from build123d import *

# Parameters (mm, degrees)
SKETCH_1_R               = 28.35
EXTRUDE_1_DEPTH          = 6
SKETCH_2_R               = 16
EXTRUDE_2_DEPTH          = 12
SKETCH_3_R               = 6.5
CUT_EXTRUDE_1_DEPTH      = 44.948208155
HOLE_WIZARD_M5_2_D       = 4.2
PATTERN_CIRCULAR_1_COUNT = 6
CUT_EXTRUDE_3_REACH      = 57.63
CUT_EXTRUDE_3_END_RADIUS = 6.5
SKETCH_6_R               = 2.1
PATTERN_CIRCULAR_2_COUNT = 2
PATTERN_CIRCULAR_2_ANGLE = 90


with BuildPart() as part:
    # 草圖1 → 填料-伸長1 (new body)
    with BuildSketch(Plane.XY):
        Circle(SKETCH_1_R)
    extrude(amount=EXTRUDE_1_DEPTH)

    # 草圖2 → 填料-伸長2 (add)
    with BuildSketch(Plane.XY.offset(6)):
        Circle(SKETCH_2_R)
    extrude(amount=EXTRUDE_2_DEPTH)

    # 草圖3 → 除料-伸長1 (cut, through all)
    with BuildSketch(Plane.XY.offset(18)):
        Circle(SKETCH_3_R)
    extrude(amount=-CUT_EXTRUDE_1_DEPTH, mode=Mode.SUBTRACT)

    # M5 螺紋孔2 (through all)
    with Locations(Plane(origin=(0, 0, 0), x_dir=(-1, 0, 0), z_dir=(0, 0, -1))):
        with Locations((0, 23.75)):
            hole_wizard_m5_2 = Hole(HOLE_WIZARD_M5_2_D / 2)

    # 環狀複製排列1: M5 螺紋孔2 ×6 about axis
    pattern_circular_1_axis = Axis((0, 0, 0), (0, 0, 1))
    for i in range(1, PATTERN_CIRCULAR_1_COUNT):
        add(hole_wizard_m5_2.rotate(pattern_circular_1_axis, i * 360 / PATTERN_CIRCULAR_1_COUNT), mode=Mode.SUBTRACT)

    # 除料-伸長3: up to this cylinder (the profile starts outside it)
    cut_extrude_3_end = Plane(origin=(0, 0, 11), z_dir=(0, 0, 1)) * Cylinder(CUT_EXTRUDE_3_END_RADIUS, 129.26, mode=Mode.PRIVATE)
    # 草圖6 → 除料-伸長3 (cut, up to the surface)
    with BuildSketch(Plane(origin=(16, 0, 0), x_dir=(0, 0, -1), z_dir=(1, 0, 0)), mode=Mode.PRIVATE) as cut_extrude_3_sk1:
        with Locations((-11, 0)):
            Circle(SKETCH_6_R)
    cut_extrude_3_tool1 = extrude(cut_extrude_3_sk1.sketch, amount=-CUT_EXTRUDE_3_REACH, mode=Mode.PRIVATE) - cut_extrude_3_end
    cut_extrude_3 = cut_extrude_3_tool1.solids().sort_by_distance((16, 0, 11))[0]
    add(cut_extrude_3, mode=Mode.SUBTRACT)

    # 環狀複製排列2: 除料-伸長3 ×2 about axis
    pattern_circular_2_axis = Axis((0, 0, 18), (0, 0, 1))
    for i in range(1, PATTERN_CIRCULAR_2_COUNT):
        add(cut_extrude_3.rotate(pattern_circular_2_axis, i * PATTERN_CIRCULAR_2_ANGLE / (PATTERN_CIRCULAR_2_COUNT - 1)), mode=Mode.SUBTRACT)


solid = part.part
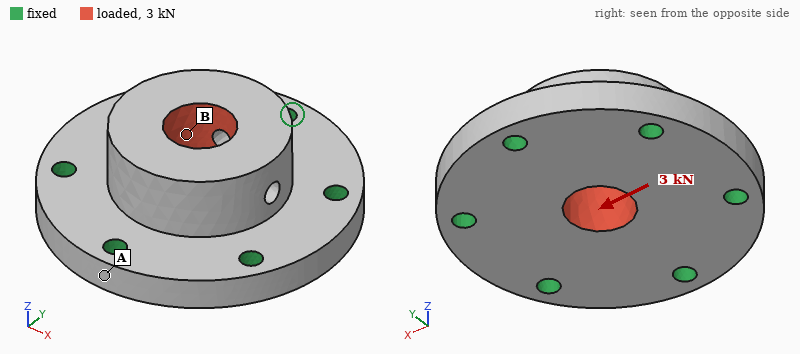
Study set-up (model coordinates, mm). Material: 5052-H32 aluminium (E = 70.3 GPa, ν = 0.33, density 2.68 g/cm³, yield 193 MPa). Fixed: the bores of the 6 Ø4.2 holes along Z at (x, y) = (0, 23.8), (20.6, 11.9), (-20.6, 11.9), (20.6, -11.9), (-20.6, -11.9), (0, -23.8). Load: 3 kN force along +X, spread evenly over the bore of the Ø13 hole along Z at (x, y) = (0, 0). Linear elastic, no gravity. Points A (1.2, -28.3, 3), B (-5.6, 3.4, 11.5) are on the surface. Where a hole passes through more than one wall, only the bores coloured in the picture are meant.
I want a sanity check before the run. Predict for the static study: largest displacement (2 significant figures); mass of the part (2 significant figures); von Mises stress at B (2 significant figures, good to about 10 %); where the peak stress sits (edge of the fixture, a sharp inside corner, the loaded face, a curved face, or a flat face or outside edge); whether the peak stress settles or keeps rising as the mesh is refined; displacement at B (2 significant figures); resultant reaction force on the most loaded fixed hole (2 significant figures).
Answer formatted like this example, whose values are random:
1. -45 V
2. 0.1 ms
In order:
1. 4.8 µm
2. 58 g
3. 5.9 MPa
4. edge of the fixture
5. keeps rising
6. 3.4 µm
7. 710 N
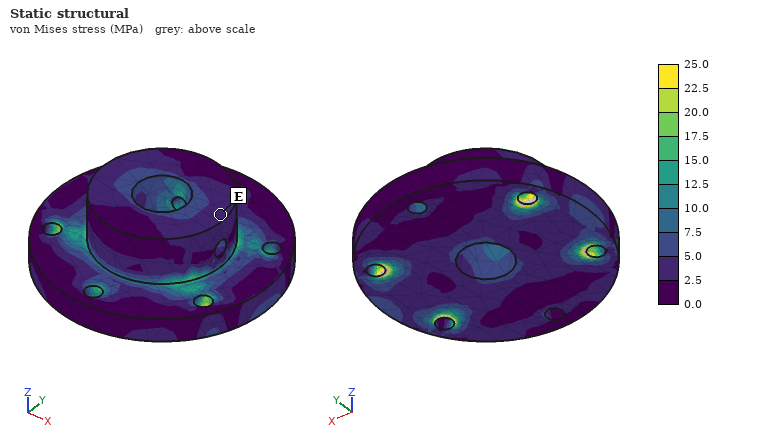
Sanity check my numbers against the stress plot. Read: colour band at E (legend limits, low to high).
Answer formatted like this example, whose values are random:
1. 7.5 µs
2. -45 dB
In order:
1. 2.5 to 5.0 MPa
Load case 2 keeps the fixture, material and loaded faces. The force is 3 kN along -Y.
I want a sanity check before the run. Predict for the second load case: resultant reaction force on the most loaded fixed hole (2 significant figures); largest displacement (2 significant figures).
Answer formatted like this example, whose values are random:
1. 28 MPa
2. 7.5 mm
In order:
1. 800 N
2. 4.8 µm
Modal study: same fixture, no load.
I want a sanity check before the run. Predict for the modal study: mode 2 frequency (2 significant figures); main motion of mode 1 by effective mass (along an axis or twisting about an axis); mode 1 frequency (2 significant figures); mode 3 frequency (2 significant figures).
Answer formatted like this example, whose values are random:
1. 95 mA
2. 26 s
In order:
1. 24 kHz
2. along Z
3. 21 kHz
4. 24 kHz
